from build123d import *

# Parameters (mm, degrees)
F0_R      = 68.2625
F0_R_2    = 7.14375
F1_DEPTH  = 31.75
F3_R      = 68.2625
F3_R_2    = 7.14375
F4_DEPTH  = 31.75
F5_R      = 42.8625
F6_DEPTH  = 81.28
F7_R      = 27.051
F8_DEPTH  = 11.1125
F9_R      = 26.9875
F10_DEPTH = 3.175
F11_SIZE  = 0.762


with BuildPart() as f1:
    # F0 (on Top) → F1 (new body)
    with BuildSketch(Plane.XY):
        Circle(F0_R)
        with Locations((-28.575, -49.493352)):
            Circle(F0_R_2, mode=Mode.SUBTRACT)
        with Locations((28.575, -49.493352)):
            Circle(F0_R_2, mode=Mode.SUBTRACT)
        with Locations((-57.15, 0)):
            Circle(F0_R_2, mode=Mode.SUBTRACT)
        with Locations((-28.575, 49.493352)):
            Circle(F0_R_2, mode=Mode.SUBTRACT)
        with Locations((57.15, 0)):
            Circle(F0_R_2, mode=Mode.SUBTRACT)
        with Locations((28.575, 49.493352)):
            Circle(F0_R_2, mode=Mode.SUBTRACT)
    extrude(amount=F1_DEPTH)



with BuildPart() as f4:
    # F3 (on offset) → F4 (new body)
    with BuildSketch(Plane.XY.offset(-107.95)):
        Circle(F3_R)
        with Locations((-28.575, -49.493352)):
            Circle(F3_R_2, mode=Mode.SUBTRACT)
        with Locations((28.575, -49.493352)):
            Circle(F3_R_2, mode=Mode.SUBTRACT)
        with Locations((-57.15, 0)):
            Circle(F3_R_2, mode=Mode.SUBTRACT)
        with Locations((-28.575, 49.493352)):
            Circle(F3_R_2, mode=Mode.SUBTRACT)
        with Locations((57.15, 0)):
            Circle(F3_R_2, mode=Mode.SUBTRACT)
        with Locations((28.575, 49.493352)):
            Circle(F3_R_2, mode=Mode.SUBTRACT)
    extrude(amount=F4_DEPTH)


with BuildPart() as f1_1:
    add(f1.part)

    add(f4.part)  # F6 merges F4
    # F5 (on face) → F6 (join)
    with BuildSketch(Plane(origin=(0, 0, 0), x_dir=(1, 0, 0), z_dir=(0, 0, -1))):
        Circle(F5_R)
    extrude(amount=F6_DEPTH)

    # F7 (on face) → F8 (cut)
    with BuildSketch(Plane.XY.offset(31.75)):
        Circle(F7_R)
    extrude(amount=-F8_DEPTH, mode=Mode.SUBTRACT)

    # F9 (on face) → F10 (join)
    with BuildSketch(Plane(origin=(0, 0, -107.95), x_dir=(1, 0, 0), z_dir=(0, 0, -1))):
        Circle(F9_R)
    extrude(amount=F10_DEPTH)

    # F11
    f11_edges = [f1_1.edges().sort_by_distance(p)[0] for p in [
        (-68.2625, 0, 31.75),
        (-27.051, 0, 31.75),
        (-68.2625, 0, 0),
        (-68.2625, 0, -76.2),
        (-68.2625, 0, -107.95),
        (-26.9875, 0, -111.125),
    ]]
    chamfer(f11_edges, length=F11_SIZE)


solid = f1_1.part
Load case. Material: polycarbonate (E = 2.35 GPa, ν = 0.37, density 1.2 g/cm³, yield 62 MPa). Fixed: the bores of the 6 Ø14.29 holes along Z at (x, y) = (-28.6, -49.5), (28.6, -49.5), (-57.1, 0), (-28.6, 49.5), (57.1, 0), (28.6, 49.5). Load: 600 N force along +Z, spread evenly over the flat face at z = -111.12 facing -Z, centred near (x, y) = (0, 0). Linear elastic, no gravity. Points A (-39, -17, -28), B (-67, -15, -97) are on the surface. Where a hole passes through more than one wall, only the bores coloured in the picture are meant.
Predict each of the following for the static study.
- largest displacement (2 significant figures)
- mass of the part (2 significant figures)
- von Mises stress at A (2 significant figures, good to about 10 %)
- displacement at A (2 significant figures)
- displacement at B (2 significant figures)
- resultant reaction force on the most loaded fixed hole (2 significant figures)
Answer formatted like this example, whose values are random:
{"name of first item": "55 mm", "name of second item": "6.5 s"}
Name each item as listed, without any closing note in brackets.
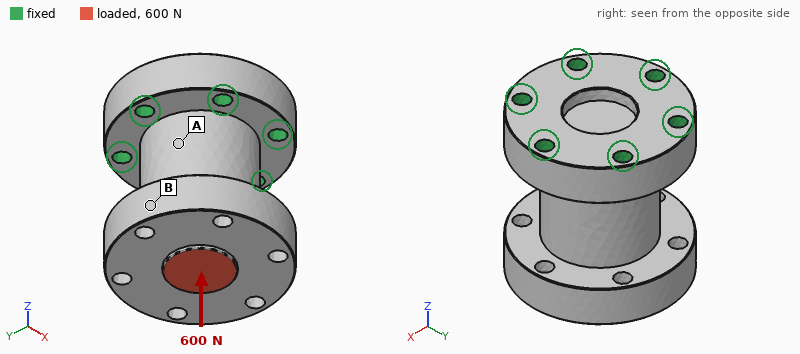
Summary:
{"largest displacement": "9.2 µm", "mass of the part": "1.5 kg", "von Mises stress at A": "0.11 MPa", "displacement at A": "3.7 µm", "displacement at B": "5.4 µm", "resultant reaction force on the most loaded fixed hole": "110 N"}
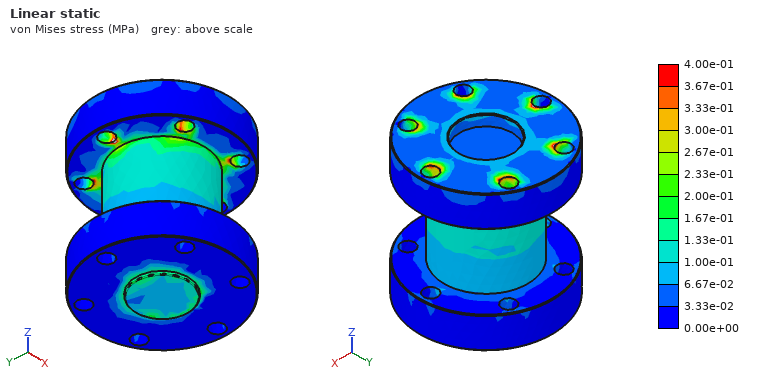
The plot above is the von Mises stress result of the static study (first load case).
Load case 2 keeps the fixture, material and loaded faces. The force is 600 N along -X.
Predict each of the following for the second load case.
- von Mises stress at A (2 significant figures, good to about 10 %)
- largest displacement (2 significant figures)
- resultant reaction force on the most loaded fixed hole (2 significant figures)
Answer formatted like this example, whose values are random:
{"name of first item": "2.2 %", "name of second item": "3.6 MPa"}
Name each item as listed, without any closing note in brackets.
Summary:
{"von Mises stress at A": "0.75 MPa", "largest displacement": "0.10 mm", "resultant reaction force on the most loaded fixed hole": "520 N"}
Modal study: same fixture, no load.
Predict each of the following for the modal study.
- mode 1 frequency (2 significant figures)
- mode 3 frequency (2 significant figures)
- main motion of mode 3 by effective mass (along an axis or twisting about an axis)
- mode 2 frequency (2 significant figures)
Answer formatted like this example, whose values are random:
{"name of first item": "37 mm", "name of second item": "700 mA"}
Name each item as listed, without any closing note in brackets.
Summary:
{"mode 1 frequency": "600 Hz", "mode 3 frequency": "940 Hz", "main motion of mode 3 by effective mass": "twisting about Z", "mode 2 frequency": "600 Hz"}
